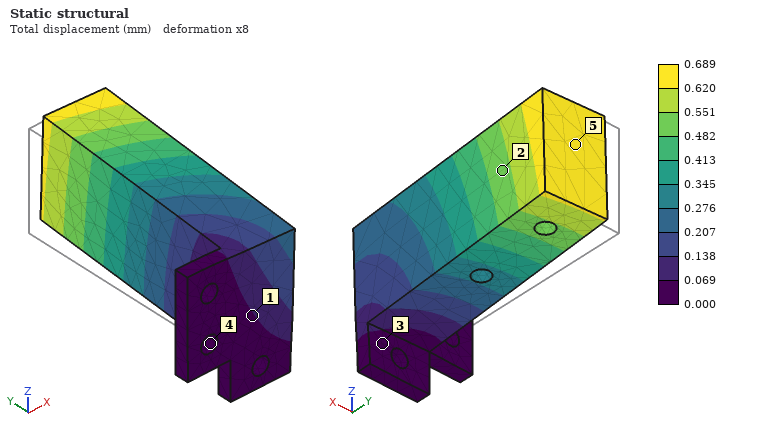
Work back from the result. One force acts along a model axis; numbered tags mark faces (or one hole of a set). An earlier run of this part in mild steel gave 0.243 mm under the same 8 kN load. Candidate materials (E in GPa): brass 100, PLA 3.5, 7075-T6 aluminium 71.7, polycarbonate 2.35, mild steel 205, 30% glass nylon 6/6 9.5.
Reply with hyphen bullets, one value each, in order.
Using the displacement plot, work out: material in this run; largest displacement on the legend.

- 7075-T6 aluminium
- 0.689 mm
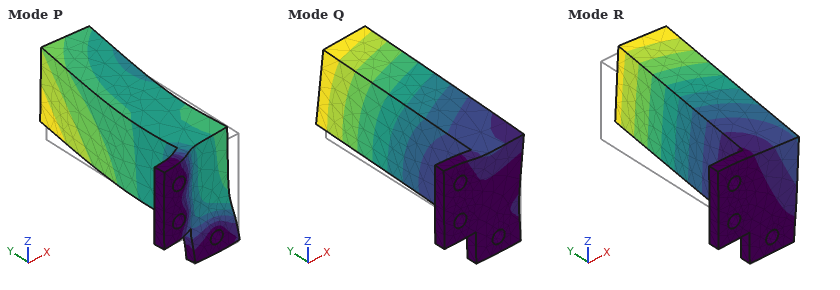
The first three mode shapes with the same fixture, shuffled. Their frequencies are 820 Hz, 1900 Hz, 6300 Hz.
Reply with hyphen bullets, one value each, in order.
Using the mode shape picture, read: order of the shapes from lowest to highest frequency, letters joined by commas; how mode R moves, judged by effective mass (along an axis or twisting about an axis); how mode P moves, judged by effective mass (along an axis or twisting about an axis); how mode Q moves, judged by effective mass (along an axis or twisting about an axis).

- R, Q, P
- along X
- along Y
- along Z
